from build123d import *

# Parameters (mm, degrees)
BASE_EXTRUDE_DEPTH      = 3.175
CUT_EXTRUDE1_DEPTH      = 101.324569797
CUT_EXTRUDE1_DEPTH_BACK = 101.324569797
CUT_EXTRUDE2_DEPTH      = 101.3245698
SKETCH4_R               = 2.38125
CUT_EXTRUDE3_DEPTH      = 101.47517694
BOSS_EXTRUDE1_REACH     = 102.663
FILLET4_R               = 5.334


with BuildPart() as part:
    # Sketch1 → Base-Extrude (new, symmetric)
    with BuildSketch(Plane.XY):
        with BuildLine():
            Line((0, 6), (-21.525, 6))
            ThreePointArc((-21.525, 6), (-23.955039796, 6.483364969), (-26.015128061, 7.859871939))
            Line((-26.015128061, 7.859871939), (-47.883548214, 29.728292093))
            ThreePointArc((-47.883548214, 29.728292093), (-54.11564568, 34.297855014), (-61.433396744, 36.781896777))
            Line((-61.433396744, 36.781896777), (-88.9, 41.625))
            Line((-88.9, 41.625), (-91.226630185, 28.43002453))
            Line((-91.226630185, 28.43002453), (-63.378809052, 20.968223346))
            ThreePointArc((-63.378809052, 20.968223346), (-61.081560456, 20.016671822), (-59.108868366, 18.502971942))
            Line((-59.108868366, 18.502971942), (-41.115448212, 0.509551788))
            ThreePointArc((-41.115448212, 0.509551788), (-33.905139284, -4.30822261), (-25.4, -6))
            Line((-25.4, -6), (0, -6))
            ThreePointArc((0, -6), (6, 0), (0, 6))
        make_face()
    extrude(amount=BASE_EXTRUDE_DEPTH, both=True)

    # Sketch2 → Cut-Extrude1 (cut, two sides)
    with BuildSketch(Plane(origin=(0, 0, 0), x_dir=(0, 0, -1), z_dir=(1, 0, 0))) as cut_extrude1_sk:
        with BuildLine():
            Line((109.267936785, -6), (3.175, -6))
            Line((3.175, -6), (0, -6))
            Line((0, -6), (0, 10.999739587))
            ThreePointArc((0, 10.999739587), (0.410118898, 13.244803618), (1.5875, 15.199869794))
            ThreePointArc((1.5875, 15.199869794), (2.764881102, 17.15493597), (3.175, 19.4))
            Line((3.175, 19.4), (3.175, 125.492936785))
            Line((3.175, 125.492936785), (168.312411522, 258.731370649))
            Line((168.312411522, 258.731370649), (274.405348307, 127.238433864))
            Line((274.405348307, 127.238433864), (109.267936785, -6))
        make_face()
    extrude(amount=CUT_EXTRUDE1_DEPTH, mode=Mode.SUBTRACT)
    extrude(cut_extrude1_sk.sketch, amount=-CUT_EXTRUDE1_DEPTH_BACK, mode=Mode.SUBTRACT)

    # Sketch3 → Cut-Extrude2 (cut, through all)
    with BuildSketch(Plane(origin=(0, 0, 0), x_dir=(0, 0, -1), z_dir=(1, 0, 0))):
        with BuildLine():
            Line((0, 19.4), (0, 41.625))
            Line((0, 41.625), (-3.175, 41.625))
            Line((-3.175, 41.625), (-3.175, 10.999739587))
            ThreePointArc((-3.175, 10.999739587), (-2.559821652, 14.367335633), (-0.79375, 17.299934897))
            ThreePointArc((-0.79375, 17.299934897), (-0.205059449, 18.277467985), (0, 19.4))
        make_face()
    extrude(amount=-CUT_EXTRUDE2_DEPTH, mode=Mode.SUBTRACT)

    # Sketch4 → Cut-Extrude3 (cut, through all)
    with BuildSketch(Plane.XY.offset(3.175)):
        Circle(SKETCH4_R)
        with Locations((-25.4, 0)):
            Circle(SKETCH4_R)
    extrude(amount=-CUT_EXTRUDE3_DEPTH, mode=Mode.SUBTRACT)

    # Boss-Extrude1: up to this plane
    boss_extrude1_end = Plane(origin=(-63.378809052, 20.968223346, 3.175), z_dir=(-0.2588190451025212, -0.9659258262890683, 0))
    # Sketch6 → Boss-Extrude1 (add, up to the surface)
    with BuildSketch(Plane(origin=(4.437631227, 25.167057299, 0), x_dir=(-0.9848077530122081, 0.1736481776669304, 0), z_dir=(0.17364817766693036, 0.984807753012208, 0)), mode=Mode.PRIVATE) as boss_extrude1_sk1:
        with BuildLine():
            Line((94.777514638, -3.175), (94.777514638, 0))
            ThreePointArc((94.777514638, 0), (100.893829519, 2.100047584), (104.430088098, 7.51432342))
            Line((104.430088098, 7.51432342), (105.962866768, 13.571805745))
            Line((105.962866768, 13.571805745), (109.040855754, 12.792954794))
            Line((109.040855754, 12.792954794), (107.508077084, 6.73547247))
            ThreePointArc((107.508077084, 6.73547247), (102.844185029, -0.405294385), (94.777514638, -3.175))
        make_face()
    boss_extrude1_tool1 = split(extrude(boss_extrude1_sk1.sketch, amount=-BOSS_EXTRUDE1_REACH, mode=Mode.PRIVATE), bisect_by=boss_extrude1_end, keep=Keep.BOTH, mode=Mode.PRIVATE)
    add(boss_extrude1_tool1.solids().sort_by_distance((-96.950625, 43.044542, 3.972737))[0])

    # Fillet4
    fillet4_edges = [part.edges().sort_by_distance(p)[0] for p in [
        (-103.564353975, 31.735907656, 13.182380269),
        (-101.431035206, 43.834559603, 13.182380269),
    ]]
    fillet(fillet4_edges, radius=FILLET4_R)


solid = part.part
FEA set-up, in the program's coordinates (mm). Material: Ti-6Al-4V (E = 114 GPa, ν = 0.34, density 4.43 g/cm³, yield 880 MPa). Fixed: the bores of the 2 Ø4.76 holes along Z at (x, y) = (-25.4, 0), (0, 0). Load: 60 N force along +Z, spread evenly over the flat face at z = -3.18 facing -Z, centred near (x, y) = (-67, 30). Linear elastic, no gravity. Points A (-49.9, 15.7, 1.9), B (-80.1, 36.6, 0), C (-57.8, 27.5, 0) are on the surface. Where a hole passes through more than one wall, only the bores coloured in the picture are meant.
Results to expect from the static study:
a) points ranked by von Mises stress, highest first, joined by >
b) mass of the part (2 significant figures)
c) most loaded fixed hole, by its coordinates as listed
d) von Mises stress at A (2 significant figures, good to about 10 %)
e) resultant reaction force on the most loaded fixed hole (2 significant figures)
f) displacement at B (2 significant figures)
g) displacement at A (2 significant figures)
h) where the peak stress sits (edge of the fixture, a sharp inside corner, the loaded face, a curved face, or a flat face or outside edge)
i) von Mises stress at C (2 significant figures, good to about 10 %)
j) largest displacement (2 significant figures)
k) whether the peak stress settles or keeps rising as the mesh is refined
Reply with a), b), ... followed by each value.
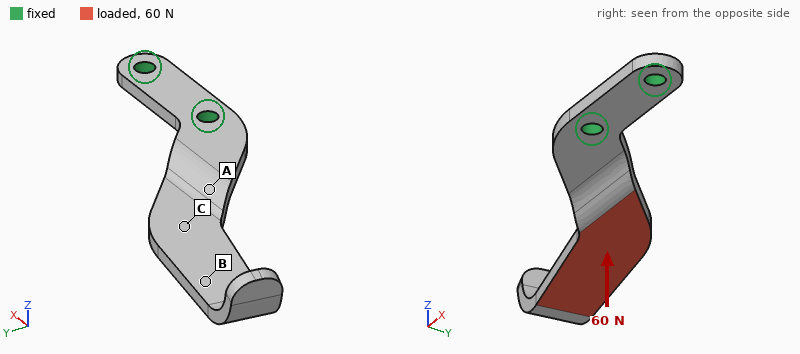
a) A > C > B
b) 25 g
c) (-25.4, 0)
d) 50 MPa
e) 65 N
f) 0.75 mm
g) 0.20 mm
h) edge of the fixture
i) 24 MPa
j) 1.1 mm
k) keeps rising
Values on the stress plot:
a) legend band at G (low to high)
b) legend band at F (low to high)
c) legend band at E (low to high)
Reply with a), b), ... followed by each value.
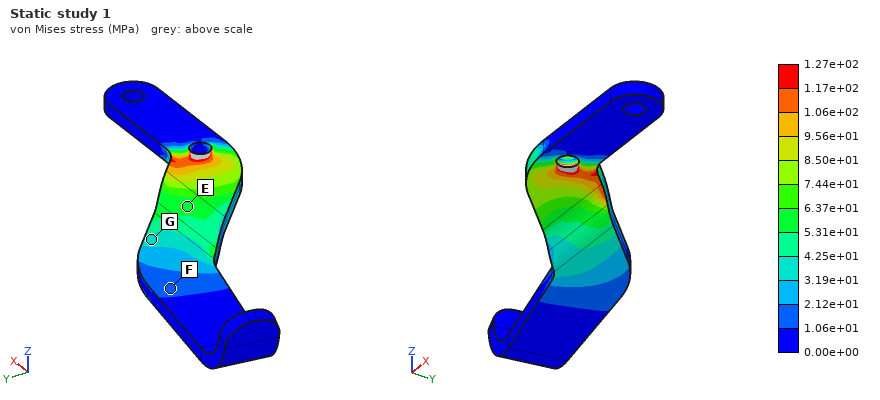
a) 3.19e+01 to 4.25e+01 MPa
b) 1.06e+01 to 2.12e+01 MPa
c) 5.31e+01 to 6.37e+01 MPa
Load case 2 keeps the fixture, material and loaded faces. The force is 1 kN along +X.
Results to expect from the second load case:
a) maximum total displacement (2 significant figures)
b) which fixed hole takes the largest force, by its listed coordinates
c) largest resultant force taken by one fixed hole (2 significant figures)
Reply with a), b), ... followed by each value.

a) 1.4 mm
b) (-25.4, 0)
c) 880 N
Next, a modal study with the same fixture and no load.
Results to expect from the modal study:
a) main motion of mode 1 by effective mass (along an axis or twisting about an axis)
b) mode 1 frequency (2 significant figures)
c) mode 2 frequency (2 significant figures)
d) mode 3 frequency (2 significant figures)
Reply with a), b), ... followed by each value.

a) along Z
b) 340 Hz
c) 1200 Hz
d) 1700 Hz
